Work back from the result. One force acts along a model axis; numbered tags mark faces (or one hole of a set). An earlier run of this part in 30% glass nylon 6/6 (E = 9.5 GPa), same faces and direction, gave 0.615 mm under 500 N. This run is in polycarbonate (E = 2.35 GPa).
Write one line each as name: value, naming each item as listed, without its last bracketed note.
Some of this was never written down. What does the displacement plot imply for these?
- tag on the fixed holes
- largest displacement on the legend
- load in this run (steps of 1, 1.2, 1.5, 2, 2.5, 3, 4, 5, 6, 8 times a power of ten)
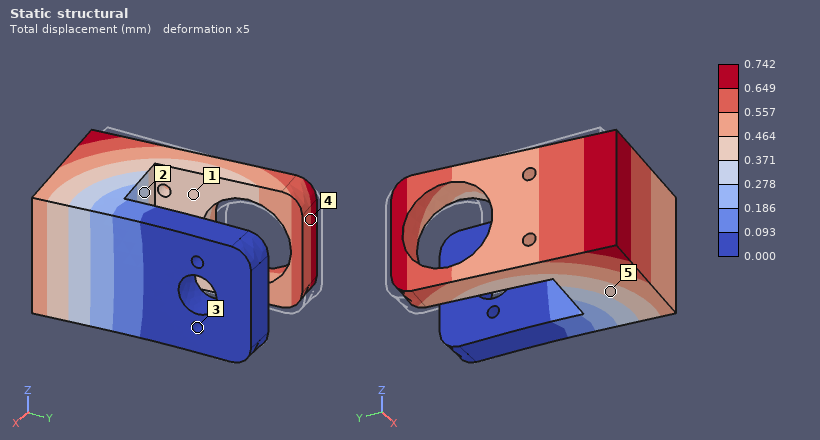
tag on the fixed holes: 3
largest displacement on the legend: 0.742 mm
load in this run: 150 N
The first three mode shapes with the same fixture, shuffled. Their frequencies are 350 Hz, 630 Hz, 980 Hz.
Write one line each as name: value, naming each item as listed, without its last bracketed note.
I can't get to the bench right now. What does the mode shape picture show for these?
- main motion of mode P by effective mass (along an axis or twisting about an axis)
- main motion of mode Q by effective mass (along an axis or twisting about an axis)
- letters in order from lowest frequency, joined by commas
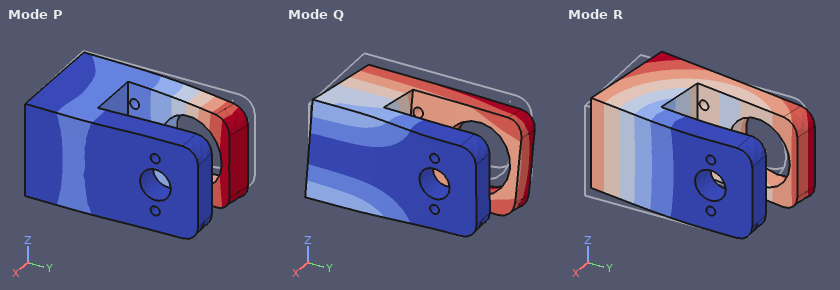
main motion of mode P by effective mass: along X
main motion of mode Q by effective mass: along Z
letters in order from lowest frequency, joined by commas: R, Q, P
